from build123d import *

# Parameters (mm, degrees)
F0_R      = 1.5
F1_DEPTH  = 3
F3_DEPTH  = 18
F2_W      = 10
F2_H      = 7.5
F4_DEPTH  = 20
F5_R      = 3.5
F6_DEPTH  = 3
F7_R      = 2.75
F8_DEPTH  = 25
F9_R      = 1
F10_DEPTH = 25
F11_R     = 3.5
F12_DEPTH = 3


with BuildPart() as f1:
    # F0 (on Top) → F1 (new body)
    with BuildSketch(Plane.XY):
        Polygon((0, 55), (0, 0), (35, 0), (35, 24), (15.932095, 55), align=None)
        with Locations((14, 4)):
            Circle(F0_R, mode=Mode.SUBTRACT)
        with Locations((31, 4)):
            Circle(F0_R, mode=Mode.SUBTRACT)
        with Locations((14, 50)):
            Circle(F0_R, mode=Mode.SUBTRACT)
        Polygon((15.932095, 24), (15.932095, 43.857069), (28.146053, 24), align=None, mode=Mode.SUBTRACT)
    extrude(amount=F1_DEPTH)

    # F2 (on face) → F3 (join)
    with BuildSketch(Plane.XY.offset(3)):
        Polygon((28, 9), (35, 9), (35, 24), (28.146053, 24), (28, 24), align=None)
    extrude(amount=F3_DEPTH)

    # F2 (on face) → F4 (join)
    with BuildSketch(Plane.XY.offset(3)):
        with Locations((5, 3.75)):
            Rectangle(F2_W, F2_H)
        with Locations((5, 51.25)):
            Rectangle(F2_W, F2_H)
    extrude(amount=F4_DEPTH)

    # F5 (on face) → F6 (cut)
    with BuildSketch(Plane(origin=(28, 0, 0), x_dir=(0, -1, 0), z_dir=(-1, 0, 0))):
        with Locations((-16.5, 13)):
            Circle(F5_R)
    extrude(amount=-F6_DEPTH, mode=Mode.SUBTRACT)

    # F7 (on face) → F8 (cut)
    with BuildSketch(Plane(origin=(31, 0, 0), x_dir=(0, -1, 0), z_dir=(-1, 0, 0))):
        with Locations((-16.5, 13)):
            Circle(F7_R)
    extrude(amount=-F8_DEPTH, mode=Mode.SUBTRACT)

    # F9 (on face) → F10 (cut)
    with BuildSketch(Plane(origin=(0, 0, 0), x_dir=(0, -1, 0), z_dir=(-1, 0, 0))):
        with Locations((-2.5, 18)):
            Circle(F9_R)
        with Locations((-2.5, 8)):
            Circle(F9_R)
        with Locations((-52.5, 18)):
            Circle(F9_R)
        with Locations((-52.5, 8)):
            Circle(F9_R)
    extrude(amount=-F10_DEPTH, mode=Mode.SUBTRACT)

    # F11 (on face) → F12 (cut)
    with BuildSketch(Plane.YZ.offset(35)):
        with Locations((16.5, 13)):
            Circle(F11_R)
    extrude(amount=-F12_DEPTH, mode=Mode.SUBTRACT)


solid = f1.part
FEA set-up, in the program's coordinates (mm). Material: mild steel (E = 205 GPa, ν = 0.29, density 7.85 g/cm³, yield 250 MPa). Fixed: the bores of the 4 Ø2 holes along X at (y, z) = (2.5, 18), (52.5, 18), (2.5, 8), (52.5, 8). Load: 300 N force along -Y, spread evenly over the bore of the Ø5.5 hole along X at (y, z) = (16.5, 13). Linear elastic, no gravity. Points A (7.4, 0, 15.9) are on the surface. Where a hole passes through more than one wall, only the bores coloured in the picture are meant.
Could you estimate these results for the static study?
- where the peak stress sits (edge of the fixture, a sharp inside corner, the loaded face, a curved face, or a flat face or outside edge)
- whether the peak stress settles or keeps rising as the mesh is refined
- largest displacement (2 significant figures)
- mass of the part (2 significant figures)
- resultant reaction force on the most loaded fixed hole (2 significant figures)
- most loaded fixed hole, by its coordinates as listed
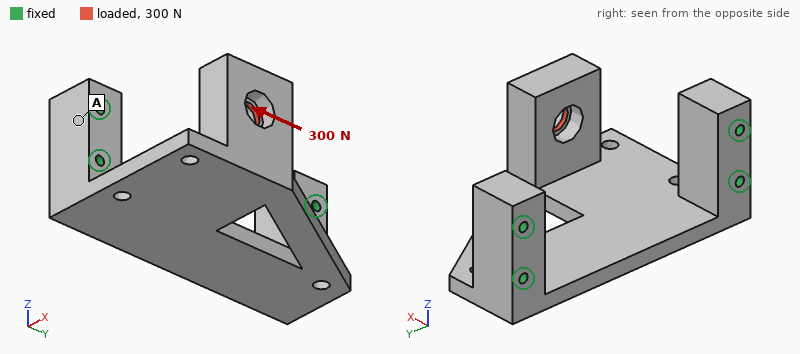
a sharp inside corner
keeps rising
55 µm
70 g
310 N
(2.5, 8)
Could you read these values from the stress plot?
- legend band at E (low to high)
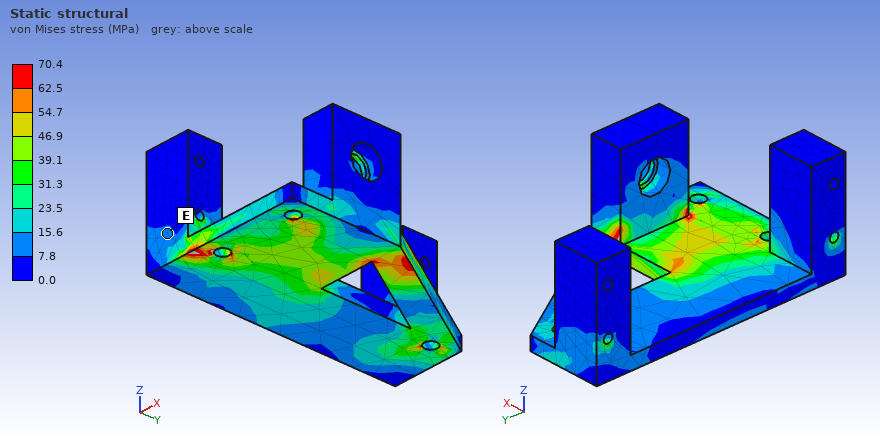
7.8 to 15.6 MPa
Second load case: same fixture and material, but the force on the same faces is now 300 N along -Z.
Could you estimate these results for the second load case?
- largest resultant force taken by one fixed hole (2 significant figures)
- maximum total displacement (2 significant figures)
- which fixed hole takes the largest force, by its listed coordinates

190 N
0.21 mm
(2.5, 8)
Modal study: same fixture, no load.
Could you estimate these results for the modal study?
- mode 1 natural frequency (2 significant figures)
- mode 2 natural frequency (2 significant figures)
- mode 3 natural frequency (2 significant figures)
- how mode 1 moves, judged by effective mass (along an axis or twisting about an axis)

1500 Hz
3500 Hz
5100 Hz
along Z
